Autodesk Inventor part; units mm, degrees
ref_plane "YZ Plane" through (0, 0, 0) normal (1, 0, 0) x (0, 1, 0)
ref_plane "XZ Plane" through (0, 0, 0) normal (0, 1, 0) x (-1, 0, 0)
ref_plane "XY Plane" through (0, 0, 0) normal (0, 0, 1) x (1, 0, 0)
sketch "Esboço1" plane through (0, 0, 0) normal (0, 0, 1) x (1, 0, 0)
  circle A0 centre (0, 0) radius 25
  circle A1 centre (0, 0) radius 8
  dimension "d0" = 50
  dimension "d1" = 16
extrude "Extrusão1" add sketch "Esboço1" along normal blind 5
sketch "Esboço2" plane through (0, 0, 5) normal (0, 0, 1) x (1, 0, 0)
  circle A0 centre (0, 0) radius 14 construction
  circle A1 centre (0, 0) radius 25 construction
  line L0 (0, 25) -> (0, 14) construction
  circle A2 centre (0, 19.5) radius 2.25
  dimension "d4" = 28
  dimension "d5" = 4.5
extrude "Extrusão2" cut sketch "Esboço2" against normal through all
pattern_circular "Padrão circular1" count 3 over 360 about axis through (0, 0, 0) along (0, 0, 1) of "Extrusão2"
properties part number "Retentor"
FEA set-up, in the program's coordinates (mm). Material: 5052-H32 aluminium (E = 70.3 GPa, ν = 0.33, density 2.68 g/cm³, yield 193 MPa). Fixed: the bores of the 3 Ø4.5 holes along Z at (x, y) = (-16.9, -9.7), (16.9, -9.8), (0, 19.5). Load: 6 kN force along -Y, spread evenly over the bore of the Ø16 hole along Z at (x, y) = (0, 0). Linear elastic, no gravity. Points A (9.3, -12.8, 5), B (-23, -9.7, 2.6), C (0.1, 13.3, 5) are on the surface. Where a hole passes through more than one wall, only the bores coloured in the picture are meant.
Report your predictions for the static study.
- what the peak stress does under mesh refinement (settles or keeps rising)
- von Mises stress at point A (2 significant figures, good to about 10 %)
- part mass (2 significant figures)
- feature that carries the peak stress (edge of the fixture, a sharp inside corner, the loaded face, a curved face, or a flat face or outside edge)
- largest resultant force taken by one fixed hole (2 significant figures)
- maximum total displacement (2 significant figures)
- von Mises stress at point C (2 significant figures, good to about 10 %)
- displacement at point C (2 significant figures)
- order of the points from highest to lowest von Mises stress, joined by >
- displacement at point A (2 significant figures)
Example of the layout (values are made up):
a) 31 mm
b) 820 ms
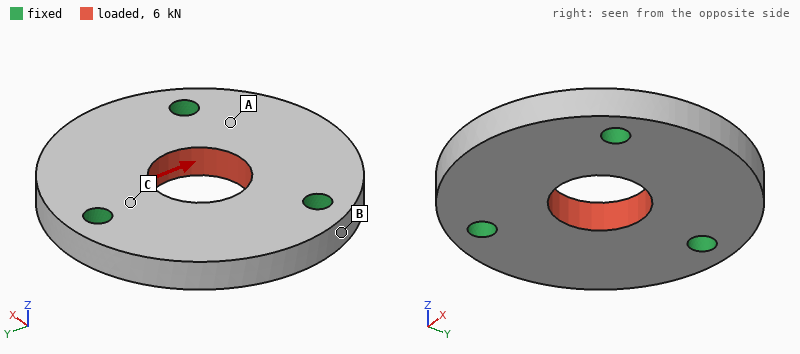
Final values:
a) keeps rising
b) 23 MPa
c) 23 g
d) edge of the fixture
e) 2.1 kN
f) 11 µm
g) 39 MPa
h) 2.3 µm
i) C > A > B
j) 5.6 µm
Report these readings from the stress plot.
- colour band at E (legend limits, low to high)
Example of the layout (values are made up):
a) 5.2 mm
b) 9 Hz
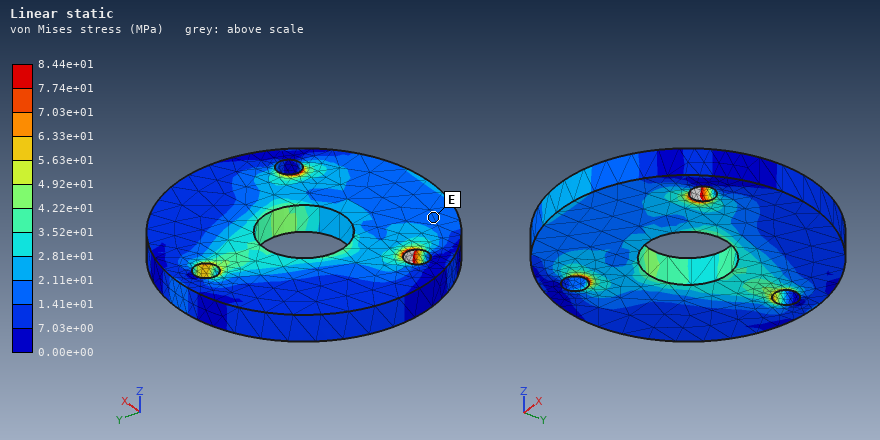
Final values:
a) 1.41e+01 to 2.11e+01 MPa
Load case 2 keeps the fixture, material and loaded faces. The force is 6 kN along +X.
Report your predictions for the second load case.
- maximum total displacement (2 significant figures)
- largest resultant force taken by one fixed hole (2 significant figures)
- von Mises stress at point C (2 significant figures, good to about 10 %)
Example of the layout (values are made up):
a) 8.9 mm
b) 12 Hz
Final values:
a) 9.9 µm
b) 2.1 kN
c) 18 MPa
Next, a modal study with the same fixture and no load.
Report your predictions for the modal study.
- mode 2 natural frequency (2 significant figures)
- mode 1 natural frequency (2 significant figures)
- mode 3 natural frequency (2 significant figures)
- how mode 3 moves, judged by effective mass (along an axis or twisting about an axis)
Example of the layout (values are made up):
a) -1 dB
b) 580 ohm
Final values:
a) 14 kHz
b) 14 kHz
c) 15 kHz
d) along Z
